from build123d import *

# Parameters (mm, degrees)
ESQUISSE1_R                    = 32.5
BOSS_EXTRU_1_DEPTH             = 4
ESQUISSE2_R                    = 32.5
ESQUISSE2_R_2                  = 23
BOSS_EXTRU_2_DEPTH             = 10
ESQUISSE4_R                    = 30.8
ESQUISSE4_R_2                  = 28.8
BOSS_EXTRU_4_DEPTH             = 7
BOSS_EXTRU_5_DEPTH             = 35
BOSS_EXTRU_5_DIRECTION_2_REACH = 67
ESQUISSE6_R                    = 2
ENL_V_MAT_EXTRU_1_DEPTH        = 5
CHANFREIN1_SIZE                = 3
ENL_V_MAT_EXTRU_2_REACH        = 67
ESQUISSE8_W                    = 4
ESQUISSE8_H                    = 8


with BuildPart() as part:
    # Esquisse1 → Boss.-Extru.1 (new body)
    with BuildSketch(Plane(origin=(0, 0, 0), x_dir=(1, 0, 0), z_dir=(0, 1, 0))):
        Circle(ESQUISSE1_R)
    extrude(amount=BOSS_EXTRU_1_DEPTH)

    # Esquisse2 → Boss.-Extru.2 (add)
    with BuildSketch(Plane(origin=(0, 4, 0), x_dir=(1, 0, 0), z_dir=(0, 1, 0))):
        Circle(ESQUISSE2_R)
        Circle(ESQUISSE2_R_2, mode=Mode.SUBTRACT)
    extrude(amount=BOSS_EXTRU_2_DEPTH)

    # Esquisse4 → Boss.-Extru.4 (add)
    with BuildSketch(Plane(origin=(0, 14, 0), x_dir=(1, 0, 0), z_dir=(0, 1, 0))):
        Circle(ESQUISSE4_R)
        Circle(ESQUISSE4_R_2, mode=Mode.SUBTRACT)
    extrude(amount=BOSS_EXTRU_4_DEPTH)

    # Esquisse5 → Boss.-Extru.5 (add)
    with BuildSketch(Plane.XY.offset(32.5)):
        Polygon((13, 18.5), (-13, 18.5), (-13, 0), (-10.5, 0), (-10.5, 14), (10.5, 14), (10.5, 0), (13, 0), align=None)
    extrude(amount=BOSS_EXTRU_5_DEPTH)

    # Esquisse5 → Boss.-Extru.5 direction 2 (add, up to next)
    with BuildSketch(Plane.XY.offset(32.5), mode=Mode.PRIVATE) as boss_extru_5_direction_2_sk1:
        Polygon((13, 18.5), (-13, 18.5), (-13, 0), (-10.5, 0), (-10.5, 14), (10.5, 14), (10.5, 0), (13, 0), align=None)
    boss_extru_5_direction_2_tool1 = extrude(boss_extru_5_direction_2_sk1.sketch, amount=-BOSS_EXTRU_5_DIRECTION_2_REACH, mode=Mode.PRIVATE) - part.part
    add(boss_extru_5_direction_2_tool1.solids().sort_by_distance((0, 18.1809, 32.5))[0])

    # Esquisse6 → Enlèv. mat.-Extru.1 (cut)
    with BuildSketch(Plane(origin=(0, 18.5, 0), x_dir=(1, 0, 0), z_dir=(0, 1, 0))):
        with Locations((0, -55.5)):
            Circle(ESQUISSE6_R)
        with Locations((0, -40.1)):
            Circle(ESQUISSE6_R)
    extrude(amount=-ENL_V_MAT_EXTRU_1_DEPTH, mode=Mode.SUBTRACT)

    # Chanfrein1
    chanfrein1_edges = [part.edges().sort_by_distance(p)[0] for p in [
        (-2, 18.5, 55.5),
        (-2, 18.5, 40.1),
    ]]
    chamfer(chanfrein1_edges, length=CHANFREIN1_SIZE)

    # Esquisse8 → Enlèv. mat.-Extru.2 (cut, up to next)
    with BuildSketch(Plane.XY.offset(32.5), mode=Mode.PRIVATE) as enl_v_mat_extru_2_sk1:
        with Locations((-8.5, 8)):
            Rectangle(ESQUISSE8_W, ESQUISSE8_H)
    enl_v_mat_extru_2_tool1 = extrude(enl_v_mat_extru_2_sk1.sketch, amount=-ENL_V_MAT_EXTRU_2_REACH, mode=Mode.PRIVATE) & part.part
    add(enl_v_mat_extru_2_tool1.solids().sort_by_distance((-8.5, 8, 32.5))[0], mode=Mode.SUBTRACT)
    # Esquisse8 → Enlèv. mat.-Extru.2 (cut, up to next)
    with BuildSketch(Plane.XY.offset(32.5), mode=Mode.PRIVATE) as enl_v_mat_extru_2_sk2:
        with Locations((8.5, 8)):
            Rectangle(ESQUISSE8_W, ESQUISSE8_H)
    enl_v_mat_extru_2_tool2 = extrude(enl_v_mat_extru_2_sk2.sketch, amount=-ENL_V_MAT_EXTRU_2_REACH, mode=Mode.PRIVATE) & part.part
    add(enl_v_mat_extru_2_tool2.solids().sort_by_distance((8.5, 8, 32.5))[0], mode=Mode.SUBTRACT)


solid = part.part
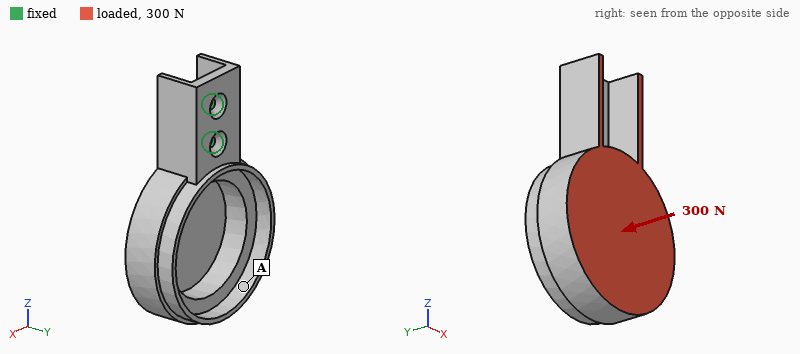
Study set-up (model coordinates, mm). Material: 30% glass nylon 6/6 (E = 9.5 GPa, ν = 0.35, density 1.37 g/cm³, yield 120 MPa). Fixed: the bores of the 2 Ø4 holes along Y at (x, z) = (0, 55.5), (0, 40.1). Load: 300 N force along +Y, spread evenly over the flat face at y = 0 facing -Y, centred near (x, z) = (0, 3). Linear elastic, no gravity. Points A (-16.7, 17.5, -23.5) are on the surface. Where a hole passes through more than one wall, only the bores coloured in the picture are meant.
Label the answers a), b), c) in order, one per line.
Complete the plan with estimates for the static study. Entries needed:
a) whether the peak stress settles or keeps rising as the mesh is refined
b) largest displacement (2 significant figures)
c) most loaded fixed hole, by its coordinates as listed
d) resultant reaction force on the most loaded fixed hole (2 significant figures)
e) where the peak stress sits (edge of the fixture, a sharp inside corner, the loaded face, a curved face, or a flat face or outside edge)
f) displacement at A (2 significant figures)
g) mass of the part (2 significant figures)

a) keeps rising
b) 1.4 mm
c) (0, 40.1)
d) 900 N
e) edge of the fixture
f) 1.2 mm
g) 53 g
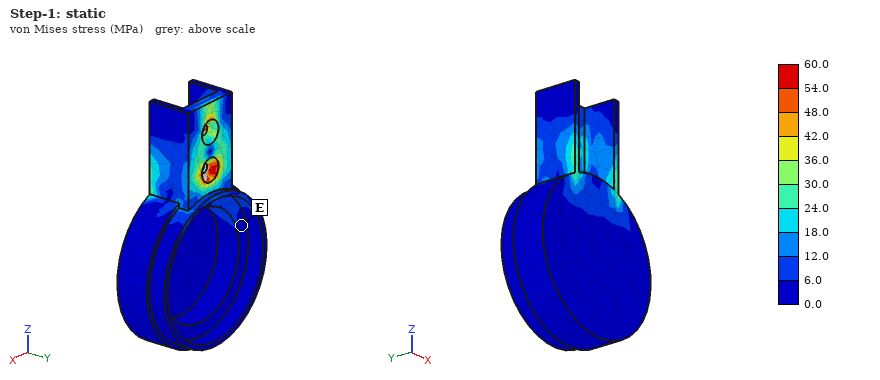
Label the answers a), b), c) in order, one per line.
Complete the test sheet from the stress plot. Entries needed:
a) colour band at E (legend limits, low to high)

a) 0.0 to 6.0 MPa
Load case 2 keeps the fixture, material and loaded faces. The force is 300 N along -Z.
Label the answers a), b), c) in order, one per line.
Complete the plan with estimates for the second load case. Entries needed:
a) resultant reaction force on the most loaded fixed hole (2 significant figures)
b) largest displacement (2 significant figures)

a) 290 N
b) 0.46 mm
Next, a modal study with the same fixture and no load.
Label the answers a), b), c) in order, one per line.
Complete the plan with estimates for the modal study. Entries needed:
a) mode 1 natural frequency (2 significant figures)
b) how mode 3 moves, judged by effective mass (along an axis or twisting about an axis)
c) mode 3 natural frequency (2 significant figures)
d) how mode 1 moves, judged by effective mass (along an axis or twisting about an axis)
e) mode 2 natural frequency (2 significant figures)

a) 410 Hz
b) along X
c) 610 Hz
d) along Y
e) 480 Hz
